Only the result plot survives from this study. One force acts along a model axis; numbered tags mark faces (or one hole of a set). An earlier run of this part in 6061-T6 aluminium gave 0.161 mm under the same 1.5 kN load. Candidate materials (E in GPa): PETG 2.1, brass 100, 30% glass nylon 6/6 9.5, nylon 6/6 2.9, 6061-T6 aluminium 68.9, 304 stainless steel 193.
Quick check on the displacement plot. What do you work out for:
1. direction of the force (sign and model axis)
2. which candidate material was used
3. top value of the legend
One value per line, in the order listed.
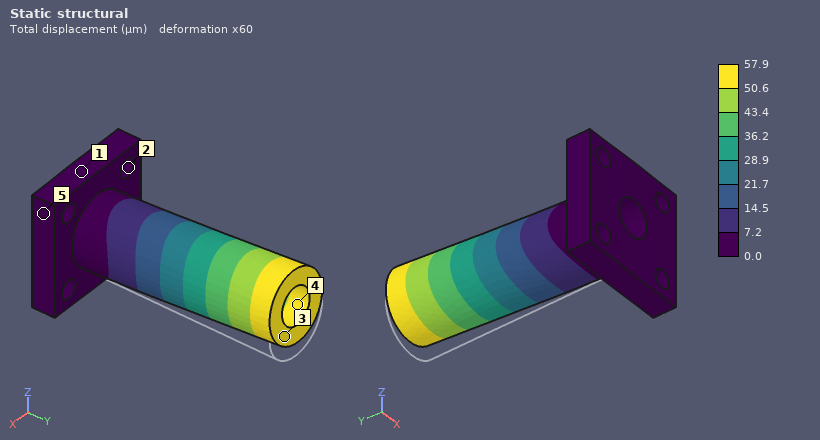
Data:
+Z
304 stainless steel
57.9 µm
